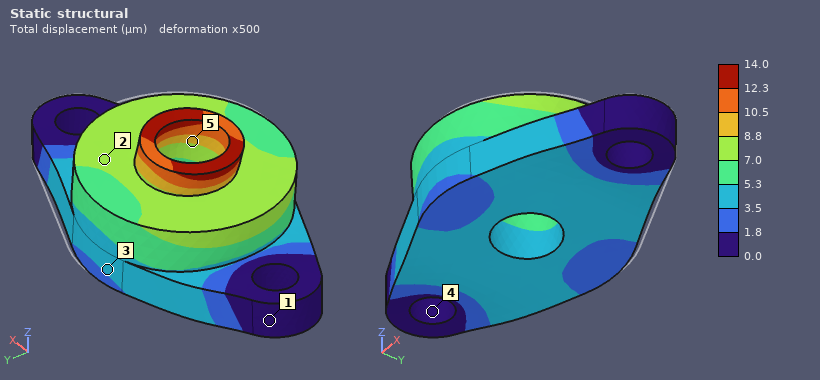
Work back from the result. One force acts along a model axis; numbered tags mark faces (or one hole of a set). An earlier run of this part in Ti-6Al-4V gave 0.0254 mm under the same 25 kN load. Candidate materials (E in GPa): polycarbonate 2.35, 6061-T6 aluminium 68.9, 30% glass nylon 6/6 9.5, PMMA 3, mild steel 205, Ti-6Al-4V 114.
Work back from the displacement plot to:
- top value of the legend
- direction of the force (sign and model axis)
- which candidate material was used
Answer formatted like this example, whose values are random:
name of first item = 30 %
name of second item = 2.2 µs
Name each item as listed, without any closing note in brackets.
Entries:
top value of the legend = 14.0 µm
direction of the force = -X
which candidate material was used = mild steel
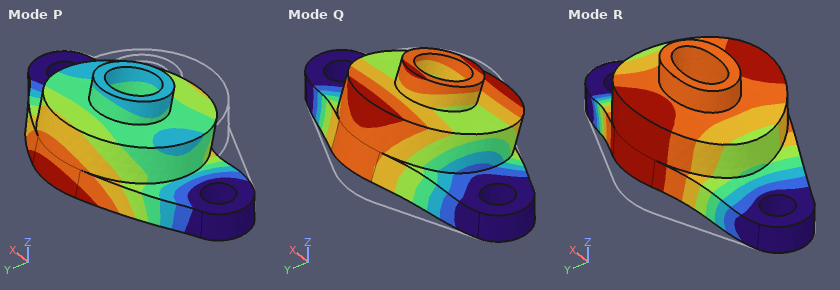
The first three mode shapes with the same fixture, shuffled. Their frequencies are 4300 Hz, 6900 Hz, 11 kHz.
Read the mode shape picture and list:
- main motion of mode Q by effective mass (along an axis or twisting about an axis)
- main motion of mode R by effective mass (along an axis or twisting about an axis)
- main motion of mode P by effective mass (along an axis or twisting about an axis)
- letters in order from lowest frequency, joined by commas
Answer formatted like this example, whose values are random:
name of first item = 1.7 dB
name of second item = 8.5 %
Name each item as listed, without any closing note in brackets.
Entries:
main motion of mode Q by effective mass = along Y
main motion of mode R by effective mass = along Z
main motion of mode P by effective mass = along Y
letters in order from lowest frequency, joined by commas = Q, R, P
